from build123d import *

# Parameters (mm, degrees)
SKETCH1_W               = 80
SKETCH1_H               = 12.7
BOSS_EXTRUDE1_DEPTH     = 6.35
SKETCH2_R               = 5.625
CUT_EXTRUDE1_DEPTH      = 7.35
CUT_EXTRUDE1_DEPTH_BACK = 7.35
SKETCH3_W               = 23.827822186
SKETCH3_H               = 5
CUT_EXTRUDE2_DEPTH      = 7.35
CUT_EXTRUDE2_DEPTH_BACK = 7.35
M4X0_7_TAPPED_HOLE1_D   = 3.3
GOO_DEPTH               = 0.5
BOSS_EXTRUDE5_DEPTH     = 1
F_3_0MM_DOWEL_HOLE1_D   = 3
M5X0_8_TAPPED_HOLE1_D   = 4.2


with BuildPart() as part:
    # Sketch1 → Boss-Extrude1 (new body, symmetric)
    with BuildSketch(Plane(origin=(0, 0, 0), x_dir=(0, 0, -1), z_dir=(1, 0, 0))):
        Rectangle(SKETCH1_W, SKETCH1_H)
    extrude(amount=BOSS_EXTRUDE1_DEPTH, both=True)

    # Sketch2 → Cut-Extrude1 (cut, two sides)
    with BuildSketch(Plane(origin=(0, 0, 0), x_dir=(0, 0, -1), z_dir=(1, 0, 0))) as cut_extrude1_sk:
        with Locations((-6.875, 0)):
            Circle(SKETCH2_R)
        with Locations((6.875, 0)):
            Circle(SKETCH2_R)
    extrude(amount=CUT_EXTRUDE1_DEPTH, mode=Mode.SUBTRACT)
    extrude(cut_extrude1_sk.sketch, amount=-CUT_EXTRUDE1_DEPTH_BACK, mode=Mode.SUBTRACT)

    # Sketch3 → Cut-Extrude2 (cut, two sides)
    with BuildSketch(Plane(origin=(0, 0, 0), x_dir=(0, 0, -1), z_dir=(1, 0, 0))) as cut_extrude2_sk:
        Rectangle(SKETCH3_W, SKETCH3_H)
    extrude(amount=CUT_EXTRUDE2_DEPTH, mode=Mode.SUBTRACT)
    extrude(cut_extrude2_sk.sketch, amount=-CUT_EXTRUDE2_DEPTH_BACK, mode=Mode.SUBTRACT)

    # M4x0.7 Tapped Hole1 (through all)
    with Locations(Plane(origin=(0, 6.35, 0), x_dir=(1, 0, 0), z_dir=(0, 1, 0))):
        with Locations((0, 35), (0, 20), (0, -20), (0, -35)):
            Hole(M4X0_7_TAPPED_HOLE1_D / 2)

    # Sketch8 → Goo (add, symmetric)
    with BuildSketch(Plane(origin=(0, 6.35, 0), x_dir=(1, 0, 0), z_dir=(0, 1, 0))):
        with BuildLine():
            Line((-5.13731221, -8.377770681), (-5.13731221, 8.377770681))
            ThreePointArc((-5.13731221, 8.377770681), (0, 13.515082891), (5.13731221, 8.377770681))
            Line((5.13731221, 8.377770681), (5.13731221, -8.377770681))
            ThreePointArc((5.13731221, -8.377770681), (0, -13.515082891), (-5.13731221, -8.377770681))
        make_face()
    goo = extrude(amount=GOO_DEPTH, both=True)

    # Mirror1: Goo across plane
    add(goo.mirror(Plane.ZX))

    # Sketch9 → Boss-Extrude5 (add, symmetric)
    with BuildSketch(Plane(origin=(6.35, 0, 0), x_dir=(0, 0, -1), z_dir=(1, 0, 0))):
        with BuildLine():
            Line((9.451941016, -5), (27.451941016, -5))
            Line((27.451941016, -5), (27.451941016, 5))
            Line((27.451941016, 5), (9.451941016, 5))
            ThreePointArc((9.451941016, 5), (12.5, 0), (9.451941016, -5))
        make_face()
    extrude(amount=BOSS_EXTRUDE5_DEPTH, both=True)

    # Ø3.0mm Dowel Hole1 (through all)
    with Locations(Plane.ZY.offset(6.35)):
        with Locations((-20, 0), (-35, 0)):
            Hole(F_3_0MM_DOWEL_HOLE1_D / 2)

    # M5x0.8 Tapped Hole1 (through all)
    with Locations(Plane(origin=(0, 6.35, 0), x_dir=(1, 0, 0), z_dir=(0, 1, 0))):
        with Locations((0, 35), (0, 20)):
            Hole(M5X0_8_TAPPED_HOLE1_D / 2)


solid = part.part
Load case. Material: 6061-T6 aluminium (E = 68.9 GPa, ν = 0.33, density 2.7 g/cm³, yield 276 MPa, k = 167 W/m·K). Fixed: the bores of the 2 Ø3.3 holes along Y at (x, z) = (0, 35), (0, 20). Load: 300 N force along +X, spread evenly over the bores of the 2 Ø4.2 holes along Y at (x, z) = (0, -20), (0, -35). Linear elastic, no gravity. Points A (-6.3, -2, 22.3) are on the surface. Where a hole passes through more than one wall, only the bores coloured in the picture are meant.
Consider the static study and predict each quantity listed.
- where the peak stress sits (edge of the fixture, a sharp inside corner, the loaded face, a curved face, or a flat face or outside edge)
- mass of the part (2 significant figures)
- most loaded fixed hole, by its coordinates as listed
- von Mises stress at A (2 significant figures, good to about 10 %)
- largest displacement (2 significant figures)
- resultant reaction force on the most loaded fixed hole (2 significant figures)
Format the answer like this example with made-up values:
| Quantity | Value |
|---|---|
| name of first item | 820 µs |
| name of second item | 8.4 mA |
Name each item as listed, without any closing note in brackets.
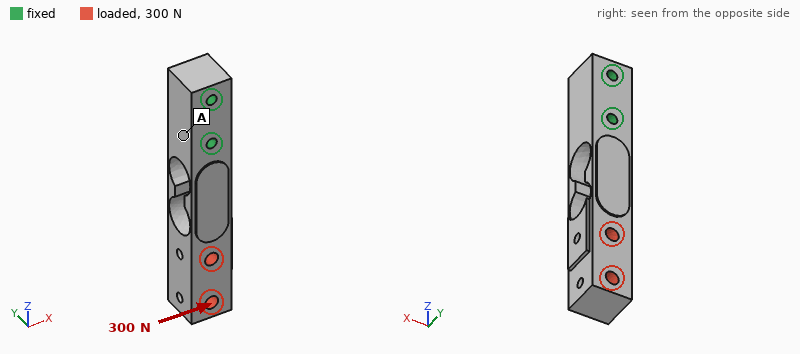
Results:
| Quantity | Value |
|---|---|
| where the peak stress sits | a curved face |
| mass of the part | 27 g |
| most loaded fixed hole, by its coordinates as listed | (0, 20) |
| von Mises stress at A | 24 MPa |
| largest displacement | 0.40 mm |
| resultant reaction force on the most loaded fixed hole | 880 N |
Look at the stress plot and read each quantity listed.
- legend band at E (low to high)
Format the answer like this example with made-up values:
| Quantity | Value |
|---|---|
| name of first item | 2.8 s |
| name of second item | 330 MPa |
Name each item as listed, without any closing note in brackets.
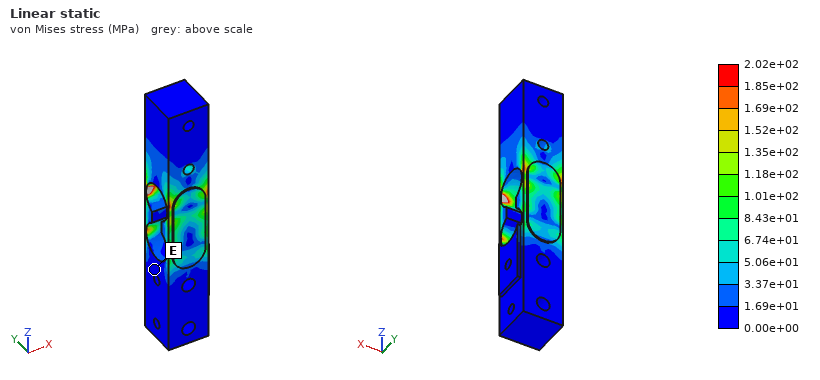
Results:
| Quantity | Value |
|---|---|
| legend band at E | 0.00e+00 to 1.69e+01 MPa |
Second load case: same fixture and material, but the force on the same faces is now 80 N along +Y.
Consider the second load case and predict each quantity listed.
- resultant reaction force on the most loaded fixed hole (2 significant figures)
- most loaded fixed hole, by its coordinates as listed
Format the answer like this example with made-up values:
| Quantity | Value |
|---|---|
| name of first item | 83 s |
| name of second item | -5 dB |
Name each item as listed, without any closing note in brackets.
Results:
| Quantity | Value |
|---|---|
| resultant reaction force on the most loaded fixed hole | 120 N |
| most loaded fixed hole, by its coordinates as listed | (0, 20) |
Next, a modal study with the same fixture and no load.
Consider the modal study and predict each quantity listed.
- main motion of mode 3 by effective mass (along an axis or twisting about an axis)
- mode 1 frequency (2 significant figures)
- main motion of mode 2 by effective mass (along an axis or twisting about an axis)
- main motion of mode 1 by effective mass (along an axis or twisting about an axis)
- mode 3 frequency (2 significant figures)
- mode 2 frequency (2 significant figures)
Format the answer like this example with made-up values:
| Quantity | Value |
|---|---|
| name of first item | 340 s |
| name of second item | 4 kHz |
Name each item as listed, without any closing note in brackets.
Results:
| Quantity | Value |
|---|---|
| main motion of mode 3 by effective mass | twisting about Z |
| mode 1 frequency | 950 Hz |
| main motion of mode 2 by effective mass | along X |
| main motion of mode 1 by effective mass | along Y |
| mode 3 frequency | 5500 Hz |
| mode 2 frequency | 1500 Hz |
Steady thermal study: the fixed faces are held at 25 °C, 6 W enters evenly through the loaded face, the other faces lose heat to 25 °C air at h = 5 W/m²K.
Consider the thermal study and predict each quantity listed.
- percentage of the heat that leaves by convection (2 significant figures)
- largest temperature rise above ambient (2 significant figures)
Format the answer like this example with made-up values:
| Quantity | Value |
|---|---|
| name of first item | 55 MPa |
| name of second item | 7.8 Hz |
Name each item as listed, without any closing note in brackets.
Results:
| Quantity | Value |
|---|---|
| percentage of the heat that leaves by convection | 5.0 % |
| largest temperature rise above ambient | 25 K |
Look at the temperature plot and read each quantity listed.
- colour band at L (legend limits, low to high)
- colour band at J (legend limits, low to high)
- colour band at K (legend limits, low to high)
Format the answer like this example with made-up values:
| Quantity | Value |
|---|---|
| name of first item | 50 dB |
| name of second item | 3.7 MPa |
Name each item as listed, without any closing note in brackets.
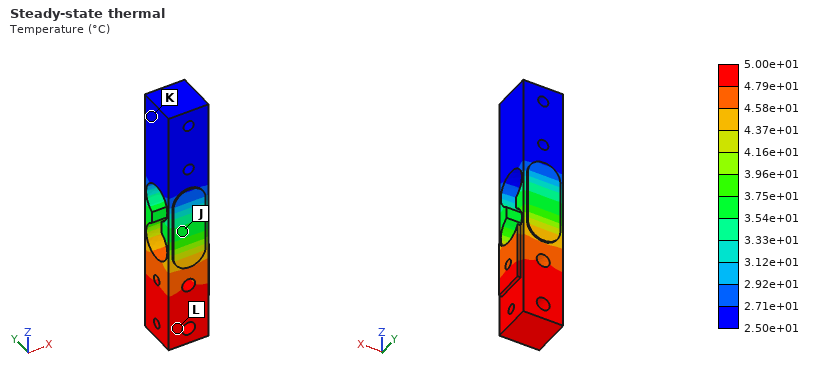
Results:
| Quantity | Value |
|---|---|
| colour band at L | 4.79e+01 to 5.00e+01 °C |
| colour band at J | 3.54e+01 to 3.75e+01 °C |
| colour band at K | 2.50e+01 to 2.71e+01 °C |
